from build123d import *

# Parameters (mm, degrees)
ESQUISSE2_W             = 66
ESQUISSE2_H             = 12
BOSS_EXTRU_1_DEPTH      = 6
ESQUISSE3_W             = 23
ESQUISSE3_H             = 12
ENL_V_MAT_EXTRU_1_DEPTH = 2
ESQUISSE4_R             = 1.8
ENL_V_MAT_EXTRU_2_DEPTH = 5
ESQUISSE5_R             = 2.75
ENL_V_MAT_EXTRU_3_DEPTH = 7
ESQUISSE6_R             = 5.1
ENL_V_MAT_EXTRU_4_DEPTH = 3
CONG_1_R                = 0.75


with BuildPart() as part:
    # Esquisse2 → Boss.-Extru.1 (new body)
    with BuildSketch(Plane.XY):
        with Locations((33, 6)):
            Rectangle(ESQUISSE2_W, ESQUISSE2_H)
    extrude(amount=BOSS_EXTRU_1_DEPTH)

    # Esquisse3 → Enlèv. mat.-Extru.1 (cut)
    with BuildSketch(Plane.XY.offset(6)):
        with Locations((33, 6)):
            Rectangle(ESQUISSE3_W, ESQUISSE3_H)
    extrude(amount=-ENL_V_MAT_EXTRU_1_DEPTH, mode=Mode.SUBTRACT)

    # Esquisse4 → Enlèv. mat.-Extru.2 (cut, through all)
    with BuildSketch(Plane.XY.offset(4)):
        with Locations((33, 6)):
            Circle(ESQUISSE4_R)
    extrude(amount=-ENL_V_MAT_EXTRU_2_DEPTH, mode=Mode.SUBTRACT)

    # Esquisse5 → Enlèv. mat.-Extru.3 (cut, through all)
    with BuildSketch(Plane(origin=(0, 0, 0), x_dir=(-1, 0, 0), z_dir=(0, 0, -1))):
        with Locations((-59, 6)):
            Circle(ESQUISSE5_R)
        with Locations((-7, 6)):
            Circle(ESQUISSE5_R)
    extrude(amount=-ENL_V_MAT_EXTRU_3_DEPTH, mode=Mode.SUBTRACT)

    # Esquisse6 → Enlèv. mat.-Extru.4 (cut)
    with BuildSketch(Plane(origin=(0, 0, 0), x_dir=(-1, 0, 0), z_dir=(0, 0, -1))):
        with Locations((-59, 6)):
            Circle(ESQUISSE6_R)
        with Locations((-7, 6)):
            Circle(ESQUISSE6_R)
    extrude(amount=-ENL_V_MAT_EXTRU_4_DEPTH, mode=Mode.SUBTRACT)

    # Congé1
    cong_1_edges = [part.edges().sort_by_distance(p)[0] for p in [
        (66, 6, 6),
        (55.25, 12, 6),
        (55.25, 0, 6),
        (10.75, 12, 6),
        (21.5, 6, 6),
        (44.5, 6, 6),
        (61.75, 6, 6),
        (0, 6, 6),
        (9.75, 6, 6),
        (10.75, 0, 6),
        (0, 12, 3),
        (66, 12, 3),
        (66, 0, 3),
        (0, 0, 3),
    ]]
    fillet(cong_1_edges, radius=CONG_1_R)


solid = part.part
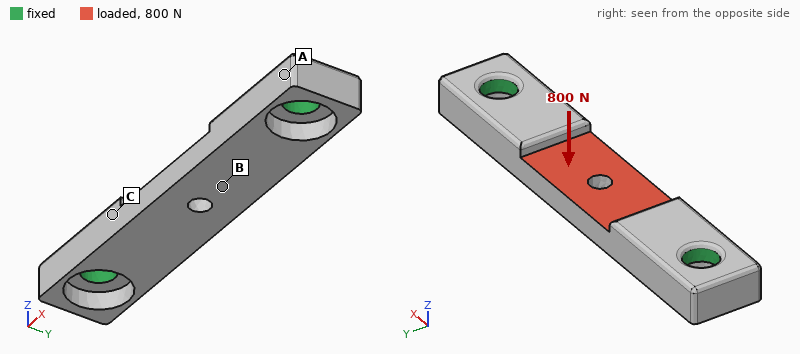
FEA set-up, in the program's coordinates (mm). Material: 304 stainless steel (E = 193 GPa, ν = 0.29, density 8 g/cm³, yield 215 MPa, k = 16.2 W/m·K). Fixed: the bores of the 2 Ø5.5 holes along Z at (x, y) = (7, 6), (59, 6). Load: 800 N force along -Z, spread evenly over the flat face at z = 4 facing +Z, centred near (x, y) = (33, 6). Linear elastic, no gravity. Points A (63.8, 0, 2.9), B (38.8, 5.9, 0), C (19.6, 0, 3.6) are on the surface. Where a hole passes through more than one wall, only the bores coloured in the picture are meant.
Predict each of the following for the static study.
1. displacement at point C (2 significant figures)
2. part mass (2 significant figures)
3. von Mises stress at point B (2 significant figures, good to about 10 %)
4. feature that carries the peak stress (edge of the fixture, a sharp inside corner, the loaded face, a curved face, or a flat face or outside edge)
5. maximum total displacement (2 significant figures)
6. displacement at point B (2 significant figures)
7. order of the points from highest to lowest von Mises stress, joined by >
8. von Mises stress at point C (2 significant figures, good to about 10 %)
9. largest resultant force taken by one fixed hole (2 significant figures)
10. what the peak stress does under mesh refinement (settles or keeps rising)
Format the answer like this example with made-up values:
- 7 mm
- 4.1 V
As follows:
- 13 µm
- 28 g
- 56 MPa
- edge of the fixture
- 28 µm
- 24 µm
- B > C > A
- 26 MPa
- 1.0 kN
- keeps rising
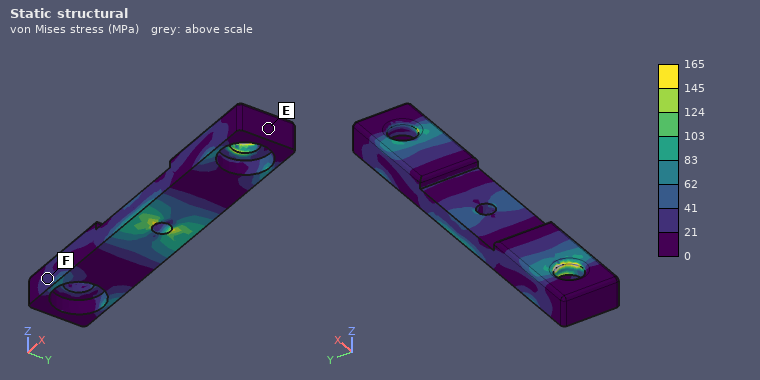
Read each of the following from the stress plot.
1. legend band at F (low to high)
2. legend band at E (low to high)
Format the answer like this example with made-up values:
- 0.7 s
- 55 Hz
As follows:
- 21 to 41 MPa
- 0 to 21 MPa
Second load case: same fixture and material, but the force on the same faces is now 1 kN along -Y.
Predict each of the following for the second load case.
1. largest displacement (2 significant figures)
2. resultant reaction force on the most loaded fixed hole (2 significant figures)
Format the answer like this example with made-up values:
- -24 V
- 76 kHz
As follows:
- 11 µm
- 500 N
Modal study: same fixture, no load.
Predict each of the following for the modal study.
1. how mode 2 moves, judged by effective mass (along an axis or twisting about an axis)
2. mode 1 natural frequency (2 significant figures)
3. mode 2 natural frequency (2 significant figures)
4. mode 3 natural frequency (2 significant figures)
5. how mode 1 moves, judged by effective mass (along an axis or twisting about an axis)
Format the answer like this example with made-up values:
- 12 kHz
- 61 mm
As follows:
- along Y
- 8900 Hz
- 15 kHz
- 18 kHz
- along Z
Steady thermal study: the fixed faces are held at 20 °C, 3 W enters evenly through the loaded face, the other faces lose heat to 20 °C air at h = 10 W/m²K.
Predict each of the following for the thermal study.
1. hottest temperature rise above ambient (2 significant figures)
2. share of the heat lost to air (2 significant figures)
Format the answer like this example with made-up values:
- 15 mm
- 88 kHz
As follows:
- 32 K
- 8.8 %
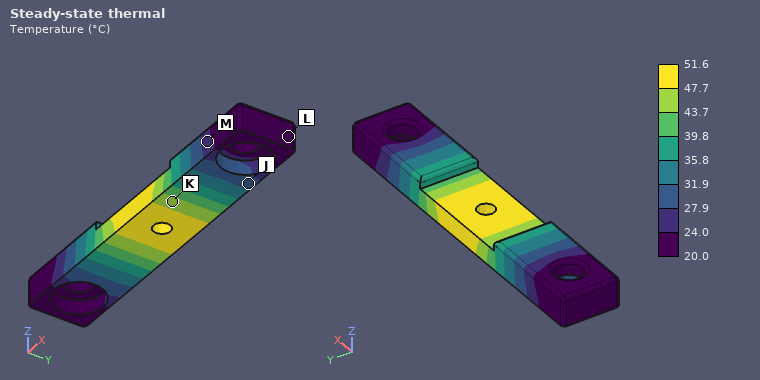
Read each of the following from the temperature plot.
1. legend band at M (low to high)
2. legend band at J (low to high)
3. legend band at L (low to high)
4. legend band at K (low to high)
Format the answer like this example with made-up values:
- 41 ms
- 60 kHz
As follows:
- 24.0 to 27.9 °C
- 27.9 to 31.9 °C
- 20.0 to 24.0 °C
- 43.7 to 47.7 °C
